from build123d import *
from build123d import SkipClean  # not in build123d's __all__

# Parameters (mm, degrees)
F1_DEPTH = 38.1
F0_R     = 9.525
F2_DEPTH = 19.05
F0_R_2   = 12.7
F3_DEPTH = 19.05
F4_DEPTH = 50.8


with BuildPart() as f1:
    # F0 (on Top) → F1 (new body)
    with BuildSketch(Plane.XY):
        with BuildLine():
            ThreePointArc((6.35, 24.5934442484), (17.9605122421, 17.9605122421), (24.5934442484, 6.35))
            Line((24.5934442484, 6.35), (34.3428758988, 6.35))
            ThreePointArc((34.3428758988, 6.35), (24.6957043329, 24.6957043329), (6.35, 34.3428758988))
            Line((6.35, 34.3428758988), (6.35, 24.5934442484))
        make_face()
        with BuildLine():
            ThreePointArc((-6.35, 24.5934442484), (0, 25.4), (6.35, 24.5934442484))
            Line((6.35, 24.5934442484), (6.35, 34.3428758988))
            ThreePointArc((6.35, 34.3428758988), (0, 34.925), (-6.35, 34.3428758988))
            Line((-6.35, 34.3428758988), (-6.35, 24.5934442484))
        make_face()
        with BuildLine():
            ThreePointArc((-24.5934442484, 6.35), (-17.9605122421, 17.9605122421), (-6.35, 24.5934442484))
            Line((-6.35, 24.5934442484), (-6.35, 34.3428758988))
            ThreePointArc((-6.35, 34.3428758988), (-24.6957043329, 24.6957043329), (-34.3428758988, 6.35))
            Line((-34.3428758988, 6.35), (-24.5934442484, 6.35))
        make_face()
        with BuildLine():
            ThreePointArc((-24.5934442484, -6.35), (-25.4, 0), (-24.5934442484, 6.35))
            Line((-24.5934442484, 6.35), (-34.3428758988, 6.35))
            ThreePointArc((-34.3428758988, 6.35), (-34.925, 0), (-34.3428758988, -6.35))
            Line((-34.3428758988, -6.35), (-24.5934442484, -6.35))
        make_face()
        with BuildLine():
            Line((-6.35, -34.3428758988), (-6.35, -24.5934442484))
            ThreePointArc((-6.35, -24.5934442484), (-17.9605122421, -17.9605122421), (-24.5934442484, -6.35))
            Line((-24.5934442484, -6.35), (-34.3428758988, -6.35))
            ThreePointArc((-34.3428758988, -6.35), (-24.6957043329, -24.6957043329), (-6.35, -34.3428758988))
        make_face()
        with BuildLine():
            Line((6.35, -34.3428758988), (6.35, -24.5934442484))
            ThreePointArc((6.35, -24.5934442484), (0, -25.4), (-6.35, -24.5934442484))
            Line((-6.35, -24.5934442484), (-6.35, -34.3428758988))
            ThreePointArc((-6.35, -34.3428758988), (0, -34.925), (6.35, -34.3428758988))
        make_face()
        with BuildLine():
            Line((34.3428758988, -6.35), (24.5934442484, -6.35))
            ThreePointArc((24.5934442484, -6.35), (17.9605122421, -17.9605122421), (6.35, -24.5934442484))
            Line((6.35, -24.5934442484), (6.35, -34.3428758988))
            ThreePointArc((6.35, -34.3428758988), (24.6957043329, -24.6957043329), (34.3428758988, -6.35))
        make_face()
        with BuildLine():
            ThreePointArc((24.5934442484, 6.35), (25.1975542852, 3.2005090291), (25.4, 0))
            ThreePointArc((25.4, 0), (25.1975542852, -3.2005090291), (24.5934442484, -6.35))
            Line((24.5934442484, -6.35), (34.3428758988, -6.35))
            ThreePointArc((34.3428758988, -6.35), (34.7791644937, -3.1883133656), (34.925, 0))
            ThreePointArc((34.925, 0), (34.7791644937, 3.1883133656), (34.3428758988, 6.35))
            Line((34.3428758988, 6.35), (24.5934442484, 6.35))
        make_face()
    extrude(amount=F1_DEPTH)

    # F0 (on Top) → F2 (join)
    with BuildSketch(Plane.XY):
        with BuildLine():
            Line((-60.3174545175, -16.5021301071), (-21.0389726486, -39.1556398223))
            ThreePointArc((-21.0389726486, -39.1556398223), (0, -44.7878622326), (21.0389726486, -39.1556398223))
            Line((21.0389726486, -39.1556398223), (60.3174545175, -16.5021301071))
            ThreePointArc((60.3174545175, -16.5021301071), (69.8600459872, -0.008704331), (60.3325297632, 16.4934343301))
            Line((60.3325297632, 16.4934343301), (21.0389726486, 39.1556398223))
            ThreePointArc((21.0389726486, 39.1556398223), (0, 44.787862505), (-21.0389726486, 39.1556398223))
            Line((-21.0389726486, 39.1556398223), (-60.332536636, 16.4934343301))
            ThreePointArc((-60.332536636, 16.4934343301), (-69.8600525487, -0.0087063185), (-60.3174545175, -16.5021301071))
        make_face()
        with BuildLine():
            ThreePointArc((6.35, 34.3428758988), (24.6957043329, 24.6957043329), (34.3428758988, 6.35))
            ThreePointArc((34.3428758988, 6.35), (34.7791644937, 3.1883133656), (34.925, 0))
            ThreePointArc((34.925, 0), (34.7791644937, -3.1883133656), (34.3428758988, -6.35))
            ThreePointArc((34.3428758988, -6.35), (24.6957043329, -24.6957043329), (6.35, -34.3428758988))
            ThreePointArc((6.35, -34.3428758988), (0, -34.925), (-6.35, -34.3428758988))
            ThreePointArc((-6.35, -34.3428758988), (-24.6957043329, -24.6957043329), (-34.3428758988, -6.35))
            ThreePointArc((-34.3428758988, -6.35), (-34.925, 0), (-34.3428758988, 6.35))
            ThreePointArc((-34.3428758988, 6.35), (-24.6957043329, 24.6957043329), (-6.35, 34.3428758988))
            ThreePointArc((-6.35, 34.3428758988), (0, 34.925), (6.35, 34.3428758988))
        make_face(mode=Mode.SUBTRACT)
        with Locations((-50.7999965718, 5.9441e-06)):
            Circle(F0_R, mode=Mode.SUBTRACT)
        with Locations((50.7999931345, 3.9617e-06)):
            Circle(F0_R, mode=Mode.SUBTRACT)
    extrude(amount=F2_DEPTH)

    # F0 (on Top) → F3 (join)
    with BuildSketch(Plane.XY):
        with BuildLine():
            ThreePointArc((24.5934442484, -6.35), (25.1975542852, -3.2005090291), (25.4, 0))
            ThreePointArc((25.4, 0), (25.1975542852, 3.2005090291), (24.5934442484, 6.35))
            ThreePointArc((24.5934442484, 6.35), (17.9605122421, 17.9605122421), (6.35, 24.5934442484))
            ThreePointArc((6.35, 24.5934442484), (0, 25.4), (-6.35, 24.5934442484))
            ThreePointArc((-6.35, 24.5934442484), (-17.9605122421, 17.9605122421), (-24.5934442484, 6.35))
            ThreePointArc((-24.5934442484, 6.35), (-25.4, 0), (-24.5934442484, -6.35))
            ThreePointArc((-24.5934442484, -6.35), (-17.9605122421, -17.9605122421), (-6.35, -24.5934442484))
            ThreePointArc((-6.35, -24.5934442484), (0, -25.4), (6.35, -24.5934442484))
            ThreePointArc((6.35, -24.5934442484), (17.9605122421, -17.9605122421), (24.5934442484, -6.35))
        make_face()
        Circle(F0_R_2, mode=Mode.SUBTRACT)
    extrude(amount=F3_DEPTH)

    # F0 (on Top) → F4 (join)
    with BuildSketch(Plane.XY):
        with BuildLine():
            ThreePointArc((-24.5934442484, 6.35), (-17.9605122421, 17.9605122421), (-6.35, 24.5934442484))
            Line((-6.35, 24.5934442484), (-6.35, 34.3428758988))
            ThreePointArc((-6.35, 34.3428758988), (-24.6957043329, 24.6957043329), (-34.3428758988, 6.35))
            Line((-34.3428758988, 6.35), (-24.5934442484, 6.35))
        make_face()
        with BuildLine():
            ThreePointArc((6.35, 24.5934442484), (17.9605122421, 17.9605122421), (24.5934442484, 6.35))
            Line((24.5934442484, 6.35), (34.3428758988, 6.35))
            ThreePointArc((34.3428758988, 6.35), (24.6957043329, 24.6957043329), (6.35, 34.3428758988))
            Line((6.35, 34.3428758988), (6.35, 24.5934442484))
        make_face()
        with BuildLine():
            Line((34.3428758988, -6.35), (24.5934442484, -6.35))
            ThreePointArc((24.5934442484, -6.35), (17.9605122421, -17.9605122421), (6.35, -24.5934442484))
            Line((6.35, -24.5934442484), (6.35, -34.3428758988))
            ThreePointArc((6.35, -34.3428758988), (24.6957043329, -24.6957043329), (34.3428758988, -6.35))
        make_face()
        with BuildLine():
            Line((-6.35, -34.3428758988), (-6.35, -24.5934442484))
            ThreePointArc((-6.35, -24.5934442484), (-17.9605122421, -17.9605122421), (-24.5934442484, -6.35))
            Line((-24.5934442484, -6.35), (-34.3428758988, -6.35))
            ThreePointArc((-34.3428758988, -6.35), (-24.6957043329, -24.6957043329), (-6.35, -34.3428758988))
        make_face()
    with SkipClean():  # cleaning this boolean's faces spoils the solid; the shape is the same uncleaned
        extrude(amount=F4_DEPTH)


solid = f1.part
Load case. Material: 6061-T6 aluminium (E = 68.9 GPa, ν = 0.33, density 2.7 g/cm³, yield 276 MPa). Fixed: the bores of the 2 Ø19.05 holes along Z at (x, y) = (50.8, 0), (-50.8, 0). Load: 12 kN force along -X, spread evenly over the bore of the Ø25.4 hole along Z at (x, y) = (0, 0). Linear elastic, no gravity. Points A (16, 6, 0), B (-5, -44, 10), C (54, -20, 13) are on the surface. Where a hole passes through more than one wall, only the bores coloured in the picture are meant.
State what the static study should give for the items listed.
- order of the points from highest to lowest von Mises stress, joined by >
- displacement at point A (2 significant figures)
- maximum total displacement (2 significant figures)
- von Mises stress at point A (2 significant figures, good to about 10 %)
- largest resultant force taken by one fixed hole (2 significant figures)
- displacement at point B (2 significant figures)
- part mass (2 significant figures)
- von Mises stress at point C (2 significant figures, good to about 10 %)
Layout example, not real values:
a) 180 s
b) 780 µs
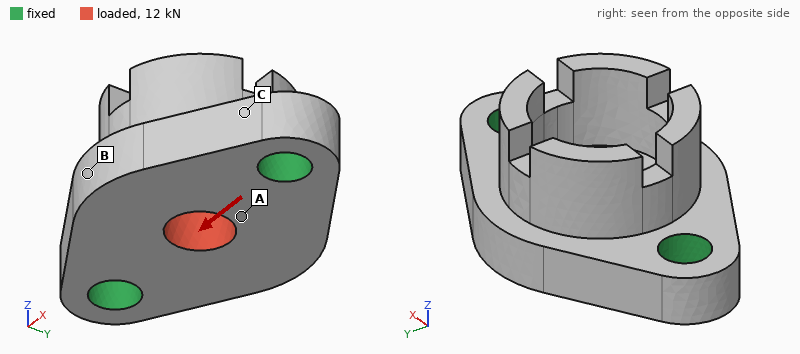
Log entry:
a) A > C > B
b) 3.6 µm
c) 4.9 µm
d) 9.7 MPa
e) 6.0 kN
f) 1.8 µm
g) 520 g
h) 3.9 MPa
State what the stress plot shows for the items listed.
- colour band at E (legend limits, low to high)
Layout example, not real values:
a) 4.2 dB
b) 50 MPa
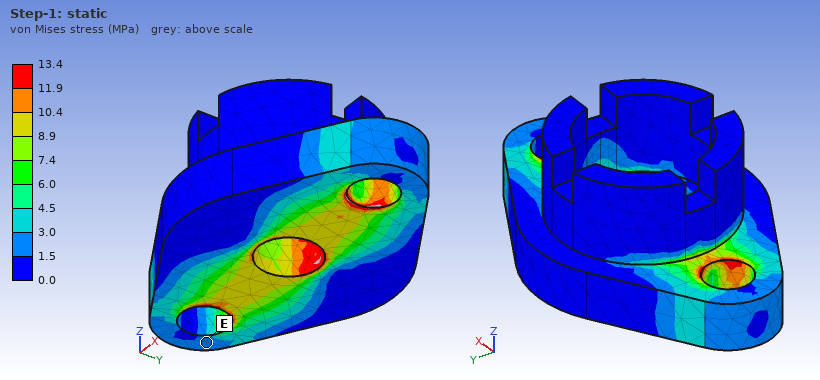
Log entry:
a) 1.5 to 3.0 MPa
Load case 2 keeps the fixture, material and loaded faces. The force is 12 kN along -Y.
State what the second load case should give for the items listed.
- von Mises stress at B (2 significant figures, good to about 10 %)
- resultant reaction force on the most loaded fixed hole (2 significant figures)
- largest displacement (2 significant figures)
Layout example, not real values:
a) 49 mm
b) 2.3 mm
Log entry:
a) 6.1 MPa
b) 6.0 kN
c) 10 µm
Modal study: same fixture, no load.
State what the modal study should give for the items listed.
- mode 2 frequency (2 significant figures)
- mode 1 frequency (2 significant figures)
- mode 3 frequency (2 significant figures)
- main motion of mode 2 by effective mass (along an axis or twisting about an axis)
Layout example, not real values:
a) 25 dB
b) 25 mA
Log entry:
a) 6400 Hz
b) 4800 Hz
c) 8700 Hz
d) along Z
